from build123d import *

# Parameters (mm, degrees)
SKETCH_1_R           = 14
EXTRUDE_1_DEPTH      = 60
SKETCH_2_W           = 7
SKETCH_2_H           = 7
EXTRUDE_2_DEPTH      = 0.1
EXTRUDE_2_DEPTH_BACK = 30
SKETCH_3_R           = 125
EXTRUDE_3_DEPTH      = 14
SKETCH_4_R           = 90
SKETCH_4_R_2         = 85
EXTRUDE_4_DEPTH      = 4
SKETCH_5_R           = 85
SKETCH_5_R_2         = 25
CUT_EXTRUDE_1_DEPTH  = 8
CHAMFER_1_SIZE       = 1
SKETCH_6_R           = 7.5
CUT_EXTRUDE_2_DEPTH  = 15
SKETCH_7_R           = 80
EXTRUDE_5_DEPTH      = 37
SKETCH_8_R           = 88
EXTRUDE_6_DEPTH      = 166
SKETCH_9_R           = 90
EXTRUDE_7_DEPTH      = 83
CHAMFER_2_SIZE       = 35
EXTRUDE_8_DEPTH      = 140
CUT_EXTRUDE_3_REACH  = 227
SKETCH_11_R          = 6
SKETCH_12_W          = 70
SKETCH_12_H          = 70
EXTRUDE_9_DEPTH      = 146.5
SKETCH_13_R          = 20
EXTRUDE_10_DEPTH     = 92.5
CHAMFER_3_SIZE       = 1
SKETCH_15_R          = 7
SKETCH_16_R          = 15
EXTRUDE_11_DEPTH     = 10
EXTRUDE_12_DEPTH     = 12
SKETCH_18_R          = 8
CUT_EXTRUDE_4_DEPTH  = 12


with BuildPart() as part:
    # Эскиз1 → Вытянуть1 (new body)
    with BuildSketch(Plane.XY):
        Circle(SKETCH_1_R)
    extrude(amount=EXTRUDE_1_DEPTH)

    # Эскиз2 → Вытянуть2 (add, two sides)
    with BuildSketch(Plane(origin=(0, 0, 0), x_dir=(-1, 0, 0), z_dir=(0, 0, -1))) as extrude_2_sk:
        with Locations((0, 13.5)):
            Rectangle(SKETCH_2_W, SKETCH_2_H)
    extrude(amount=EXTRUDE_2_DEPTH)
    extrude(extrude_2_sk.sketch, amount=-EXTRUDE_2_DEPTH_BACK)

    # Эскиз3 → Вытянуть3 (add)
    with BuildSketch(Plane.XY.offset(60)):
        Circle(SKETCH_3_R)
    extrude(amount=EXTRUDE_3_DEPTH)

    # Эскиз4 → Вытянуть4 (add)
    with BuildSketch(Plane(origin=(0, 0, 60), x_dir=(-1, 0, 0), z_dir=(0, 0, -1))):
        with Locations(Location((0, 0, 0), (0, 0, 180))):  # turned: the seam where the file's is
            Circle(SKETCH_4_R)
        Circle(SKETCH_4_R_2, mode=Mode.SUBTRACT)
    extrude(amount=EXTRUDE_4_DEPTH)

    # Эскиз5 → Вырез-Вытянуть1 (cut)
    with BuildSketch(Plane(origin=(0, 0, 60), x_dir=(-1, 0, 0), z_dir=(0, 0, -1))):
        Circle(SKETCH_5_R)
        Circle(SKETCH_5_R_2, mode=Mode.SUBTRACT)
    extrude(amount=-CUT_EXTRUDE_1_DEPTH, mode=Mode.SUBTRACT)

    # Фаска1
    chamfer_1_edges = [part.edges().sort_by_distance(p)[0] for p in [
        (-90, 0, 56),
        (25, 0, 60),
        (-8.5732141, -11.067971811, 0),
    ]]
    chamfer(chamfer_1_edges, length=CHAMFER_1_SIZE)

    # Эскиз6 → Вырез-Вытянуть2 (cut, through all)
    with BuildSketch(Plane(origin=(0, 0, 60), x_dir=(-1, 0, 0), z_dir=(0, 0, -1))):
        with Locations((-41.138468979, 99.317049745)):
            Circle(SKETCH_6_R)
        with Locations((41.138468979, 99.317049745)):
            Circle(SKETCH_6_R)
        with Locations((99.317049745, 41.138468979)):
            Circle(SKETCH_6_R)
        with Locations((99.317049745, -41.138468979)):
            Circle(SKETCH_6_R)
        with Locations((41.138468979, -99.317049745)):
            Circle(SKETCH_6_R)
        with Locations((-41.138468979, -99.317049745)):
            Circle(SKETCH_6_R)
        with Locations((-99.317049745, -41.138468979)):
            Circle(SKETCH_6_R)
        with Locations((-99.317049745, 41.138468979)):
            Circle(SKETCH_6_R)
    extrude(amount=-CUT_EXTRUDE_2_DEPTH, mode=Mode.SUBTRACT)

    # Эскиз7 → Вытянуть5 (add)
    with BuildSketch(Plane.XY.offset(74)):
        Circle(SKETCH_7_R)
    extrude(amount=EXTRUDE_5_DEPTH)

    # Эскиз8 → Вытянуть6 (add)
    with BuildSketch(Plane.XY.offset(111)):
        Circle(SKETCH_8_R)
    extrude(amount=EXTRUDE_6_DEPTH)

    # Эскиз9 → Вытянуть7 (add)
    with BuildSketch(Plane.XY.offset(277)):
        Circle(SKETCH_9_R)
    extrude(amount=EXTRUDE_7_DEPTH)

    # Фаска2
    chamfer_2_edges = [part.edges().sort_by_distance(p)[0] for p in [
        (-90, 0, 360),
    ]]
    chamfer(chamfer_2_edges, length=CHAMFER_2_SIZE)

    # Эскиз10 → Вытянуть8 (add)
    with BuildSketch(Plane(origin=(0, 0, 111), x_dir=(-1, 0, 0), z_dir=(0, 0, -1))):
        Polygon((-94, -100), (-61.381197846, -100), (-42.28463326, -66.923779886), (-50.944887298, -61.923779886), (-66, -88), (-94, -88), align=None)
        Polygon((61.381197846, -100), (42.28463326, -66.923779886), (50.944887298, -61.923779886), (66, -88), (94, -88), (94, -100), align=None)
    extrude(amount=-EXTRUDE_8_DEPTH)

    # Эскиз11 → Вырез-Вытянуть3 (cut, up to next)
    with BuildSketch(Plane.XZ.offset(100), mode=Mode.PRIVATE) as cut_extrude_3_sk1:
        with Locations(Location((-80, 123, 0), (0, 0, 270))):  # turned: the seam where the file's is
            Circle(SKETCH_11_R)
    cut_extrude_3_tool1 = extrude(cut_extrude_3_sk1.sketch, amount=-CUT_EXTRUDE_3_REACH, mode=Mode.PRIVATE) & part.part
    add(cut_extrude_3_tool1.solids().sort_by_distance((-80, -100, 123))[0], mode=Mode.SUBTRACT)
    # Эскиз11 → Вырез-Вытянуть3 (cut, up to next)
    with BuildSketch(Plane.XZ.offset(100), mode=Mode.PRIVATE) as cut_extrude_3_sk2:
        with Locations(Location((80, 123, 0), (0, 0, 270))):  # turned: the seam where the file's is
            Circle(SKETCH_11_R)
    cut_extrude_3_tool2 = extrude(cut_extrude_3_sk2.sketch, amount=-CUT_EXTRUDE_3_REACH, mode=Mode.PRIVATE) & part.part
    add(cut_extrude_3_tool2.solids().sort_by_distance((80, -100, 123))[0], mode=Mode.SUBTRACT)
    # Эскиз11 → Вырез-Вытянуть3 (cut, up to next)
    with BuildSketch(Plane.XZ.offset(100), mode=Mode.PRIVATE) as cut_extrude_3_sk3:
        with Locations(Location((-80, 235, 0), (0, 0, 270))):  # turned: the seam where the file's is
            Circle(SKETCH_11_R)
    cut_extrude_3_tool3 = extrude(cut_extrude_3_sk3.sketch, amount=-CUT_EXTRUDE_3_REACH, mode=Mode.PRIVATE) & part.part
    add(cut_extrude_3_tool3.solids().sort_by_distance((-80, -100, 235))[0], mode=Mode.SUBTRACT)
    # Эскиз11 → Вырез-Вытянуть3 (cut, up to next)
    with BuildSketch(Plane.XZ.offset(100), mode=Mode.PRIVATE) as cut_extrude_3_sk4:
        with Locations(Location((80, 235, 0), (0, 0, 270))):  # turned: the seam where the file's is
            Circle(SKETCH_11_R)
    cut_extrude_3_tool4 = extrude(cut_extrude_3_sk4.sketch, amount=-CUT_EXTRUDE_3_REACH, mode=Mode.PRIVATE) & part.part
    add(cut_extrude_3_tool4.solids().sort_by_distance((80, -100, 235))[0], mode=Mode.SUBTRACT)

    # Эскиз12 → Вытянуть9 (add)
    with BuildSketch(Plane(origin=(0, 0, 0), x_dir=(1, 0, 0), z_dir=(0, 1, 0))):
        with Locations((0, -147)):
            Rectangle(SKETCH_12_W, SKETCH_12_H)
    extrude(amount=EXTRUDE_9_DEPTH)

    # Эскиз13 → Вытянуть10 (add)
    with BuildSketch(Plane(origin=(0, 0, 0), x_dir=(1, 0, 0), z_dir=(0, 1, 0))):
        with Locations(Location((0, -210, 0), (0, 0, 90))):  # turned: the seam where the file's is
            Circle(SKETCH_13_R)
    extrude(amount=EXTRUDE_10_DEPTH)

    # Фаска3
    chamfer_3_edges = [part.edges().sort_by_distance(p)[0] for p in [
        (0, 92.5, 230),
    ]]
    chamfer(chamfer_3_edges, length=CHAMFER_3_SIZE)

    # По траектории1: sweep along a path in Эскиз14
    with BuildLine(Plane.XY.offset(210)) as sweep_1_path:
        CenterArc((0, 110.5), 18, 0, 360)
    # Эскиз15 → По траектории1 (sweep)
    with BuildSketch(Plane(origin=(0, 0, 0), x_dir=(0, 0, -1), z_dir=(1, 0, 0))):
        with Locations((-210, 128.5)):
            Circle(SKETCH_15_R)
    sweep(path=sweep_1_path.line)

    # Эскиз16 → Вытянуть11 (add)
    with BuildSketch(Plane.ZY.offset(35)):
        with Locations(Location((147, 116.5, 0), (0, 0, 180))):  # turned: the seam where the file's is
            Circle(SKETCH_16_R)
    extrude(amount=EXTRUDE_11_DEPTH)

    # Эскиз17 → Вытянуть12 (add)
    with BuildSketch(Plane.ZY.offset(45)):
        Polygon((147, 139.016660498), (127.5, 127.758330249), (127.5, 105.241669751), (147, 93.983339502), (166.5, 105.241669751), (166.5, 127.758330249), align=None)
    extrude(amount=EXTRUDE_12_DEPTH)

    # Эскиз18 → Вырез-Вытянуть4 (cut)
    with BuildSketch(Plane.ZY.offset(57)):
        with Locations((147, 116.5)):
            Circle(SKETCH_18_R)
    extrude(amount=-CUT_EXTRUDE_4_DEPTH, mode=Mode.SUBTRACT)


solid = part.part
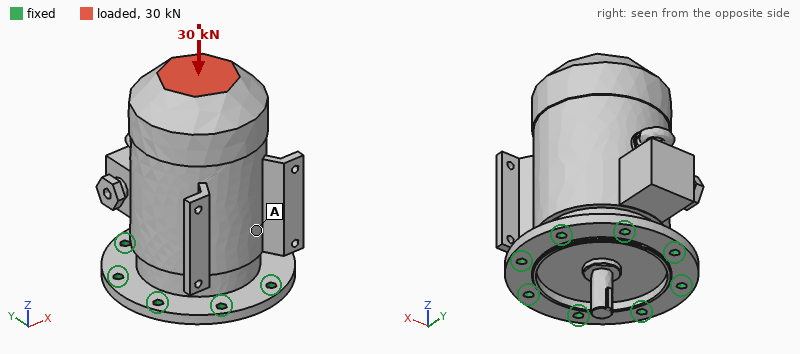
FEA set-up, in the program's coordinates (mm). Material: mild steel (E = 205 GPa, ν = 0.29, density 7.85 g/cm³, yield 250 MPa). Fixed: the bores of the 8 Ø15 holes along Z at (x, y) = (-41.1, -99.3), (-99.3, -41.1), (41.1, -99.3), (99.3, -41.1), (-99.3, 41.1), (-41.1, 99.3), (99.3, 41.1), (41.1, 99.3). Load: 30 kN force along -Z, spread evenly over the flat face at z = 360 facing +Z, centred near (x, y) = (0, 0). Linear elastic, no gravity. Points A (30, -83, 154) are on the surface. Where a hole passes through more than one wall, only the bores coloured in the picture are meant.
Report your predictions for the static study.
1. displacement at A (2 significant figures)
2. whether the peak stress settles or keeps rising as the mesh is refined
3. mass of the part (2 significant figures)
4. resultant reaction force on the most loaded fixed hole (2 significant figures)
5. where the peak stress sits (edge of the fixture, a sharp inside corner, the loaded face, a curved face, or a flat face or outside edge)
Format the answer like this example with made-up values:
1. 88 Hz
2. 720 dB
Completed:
1. 8.5 µm
2. keeps rising
3. 60 kg
4. 5.0 kN
5. edge of the fixture
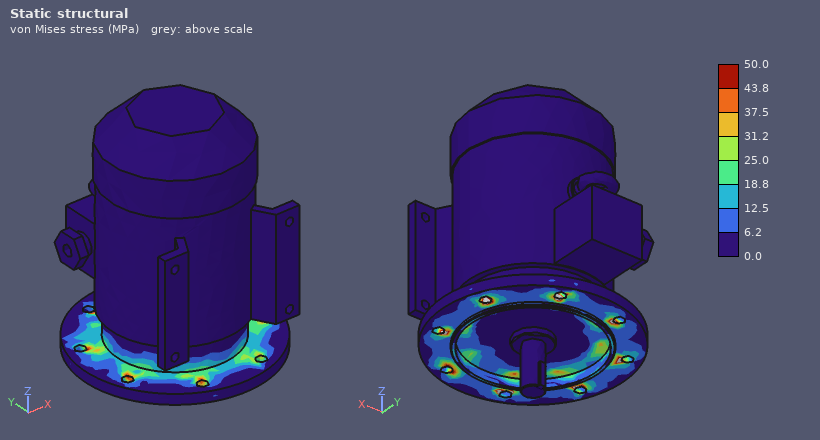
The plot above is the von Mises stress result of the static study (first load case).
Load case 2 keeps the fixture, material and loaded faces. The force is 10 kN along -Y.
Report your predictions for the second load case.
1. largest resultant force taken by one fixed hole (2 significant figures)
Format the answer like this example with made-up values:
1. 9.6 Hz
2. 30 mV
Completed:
1. 8.6 kN
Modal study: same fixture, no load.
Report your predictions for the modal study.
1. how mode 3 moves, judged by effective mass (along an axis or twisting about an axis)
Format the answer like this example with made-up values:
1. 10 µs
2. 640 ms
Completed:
1. along Z
